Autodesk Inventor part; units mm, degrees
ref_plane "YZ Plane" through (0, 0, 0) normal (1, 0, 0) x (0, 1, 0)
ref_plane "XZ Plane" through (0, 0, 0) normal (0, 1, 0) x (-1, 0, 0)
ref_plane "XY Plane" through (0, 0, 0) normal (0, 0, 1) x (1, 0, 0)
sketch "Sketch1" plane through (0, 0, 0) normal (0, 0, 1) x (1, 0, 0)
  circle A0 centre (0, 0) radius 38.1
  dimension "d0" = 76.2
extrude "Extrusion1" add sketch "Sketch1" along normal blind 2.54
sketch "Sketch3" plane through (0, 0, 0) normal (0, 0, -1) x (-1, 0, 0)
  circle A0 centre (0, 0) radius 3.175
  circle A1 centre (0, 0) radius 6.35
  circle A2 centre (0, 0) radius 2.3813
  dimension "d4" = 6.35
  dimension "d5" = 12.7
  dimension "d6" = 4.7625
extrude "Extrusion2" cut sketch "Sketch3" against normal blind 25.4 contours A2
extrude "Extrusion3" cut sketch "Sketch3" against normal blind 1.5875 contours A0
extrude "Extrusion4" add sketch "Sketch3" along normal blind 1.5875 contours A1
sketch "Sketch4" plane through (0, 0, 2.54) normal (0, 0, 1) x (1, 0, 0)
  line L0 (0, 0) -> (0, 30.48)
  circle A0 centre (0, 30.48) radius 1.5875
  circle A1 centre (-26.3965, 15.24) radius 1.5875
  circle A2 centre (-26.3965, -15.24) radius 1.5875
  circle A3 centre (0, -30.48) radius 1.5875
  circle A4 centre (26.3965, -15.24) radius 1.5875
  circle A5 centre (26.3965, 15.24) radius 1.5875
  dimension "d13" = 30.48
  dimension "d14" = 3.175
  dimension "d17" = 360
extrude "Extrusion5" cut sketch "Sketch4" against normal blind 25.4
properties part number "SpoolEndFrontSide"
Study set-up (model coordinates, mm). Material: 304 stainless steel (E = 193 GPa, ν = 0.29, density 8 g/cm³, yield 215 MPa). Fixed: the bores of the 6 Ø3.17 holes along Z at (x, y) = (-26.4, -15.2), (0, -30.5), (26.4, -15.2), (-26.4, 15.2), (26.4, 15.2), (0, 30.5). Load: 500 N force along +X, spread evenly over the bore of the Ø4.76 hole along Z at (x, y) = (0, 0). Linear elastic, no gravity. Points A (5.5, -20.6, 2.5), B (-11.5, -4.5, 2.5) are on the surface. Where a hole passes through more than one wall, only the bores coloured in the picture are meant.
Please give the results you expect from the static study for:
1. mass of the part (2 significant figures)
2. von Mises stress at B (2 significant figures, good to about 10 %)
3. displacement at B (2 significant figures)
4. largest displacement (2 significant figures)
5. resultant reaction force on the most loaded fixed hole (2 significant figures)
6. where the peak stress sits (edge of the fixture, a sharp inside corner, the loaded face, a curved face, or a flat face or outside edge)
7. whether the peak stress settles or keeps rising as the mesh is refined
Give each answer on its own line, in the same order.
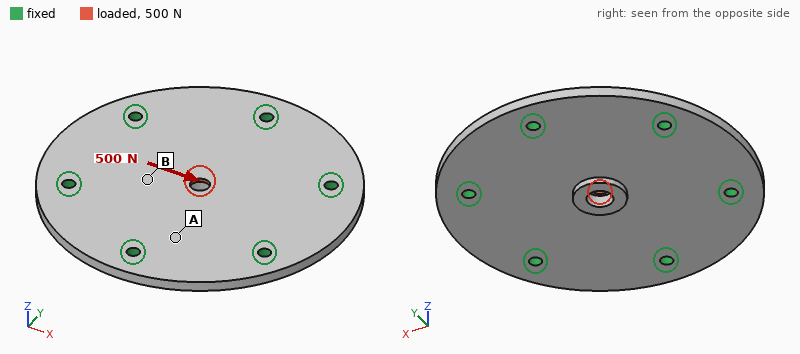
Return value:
92 g
5.7 MPa
0.69 µm
1.2 µm
110 N
a sharp inside corner
keeps rising
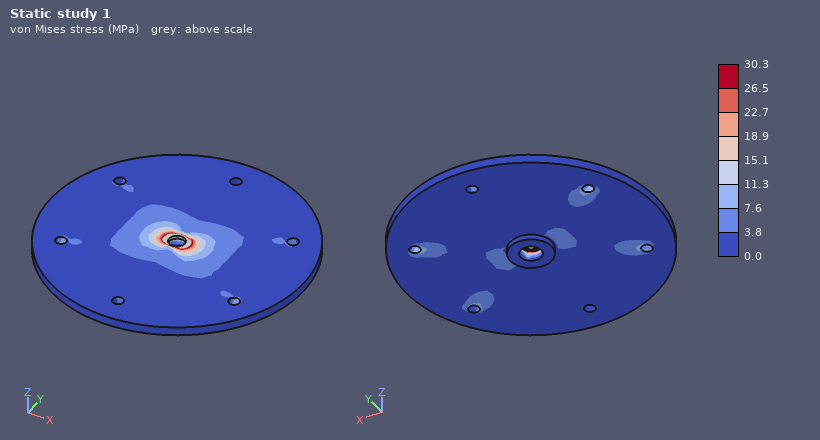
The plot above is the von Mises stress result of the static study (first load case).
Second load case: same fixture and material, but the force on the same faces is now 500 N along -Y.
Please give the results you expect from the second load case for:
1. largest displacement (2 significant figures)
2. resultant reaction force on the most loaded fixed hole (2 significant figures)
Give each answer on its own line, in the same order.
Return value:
1.2 µm
130 N
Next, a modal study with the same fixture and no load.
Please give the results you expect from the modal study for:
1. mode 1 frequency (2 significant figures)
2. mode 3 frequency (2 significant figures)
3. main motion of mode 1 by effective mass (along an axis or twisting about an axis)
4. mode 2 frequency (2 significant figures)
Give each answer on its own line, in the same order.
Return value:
5600 Hz
11 kHz
along Z
10 kHz
